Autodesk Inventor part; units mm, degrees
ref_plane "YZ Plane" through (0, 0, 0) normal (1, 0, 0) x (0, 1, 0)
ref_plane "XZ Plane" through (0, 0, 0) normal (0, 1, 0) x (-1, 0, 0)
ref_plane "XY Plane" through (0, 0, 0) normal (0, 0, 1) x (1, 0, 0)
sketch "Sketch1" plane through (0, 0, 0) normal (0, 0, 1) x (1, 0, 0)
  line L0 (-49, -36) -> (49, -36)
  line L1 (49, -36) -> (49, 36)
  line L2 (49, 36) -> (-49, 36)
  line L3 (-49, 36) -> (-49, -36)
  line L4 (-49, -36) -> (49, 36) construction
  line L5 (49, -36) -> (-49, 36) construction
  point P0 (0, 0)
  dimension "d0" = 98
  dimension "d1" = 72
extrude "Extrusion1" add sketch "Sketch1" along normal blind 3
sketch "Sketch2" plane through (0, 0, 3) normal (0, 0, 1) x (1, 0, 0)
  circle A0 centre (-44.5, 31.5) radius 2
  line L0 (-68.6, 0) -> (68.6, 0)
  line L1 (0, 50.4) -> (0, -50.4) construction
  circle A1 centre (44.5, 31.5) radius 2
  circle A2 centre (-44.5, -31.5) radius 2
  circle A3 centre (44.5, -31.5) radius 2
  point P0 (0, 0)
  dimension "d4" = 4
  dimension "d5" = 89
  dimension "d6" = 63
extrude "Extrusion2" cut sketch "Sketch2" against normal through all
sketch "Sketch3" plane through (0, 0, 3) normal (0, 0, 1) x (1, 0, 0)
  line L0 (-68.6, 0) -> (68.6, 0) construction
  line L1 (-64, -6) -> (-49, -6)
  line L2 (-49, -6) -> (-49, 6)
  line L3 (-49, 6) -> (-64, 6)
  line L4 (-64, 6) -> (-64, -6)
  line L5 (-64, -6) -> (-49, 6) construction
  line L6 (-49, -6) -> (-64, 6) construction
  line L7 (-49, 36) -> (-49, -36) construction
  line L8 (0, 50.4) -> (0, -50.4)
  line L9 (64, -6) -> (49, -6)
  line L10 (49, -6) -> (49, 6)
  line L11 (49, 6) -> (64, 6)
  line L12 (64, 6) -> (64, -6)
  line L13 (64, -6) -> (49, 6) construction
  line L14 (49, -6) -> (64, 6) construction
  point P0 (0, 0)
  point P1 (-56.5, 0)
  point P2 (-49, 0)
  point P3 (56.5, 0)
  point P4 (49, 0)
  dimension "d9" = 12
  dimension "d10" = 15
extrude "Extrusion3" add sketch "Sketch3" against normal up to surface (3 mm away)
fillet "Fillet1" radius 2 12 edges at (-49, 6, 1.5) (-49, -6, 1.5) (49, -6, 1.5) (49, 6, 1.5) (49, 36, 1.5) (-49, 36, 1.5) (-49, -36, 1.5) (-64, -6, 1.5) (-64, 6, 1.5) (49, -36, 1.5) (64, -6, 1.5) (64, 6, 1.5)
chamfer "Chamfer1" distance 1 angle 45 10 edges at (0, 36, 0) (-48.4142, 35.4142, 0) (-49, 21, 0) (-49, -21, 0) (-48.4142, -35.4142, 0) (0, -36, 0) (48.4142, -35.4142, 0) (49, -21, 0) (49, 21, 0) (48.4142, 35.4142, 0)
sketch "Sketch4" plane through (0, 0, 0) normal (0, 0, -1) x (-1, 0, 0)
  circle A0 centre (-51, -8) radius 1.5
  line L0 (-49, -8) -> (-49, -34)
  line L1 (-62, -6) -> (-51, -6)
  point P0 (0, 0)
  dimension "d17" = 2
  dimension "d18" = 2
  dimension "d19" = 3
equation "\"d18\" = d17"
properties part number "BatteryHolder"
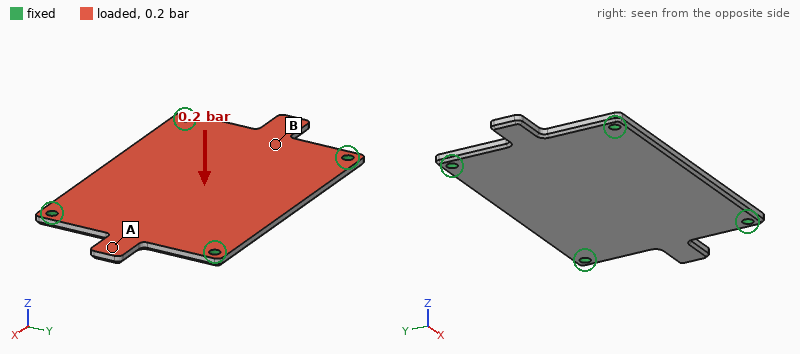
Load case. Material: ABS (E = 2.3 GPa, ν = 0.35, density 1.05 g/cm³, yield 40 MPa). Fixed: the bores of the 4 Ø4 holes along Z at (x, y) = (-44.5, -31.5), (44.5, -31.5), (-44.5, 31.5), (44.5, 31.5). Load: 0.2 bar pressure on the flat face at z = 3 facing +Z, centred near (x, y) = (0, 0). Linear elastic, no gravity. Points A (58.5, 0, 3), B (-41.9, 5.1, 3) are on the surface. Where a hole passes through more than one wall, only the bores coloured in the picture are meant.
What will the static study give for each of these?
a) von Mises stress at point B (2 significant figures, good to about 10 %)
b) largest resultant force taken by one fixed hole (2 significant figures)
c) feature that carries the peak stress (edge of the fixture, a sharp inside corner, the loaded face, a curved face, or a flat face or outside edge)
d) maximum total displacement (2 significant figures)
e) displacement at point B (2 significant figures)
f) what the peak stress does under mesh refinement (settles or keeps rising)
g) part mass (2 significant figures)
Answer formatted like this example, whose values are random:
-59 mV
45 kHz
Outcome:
3.8 MPa
37 N
edge of the fixture
1.0 mm
0.32 mm
keeps rising
23 g
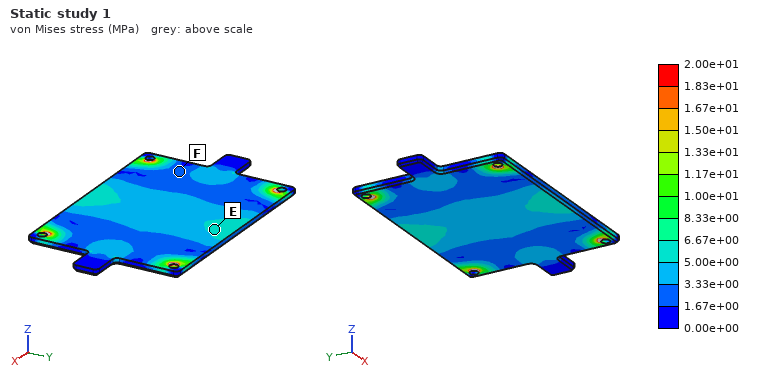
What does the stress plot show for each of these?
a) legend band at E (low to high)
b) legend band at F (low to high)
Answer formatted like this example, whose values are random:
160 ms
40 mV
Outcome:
5.00e+00 to 6.67e+00 MPa
1.67e+00 to 3.33e+00 MPa
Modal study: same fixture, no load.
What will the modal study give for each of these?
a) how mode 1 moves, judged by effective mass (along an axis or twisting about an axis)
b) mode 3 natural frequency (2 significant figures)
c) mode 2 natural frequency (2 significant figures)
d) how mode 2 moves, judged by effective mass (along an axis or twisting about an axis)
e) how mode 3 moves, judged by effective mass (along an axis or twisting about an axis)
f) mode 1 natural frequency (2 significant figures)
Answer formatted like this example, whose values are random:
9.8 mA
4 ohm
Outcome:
along Z
870 Hz
740 Hz
twisting about X
along Z
450 Hz
